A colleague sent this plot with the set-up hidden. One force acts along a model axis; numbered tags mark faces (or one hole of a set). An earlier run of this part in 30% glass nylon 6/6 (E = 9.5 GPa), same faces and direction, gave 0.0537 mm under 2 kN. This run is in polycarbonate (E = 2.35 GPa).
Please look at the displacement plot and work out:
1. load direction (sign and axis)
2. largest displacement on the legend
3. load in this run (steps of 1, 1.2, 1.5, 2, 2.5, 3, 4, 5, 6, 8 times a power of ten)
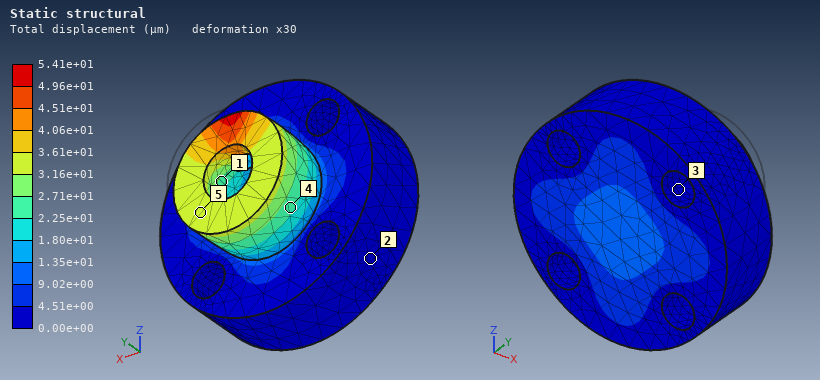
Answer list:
-Y
5.41e+01 µm
500 N
